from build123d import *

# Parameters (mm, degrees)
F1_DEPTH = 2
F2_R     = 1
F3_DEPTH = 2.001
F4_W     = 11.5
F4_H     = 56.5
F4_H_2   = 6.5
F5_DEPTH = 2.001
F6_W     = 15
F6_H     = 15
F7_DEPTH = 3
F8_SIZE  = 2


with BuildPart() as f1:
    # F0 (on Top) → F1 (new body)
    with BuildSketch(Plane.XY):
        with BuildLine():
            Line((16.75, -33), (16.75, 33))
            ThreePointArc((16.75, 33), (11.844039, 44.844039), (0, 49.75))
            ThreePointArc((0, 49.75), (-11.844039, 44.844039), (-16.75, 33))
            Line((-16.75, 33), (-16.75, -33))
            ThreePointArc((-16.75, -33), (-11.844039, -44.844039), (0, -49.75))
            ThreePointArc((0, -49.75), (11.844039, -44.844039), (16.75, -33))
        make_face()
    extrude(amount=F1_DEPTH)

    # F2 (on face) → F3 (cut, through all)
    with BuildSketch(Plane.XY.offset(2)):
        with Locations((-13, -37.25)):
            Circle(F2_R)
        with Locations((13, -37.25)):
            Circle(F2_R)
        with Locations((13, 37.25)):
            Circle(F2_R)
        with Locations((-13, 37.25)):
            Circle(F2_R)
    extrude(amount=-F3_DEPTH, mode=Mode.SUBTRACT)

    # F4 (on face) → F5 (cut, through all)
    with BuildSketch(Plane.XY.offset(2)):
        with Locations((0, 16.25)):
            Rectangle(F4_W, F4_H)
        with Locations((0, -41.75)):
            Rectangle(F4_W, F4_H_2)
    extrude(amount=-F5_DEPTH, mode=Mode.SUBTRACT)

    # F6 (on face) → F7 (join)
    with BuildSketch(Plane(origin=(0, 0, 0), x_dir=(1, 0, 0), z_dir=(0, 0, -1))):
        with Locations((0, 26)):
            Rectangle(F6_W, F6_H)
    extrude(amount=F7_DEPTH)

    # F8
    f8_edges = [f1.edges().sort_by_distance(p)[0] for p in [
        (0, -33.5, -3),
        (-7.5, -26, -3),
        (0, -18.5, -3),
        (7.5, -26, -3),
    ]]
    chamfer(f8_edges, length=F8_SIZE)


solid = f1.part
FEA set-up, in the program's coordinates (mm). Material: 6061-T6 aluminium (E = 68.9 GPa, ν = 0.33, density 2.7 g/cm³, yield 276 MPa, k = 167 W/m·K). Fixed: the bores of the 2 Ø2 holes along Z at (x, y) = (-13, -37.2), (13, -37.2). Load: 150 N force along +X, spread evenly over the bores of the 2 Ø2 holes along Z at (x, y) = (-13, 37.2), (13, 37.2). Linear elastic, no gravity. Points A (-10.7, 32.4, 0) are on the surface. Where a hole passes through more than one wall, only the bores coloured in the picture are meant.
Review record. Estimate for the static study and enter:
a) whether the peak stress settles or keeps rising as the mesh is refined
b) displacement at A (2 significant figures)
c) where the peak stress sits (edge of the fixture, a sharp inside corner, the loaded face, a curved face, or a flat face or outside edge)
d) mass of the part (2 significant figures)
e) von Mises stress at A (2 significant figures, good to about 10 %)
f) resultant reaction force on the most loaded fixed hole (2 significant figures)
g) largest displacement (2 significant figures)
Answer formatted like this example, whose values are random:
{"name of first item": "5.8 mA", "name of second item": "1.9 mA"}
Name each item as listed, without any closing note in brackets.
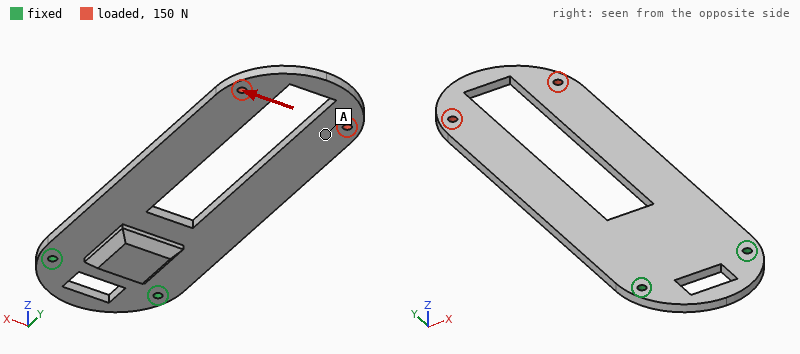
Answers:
{"whether the peak stress settles or keeps rising as the mesh is refined": "keeps rising", "displacement at A": "0.19 mm", "where the peak stress sits": "a sharp inside corner", "mass of the part": "14 g", "von Mises stress at A": "9.8 MPa", "resultant reaction force on the most loaded fixed hole": "430 N", "largest displacement": "0.24 mm"}
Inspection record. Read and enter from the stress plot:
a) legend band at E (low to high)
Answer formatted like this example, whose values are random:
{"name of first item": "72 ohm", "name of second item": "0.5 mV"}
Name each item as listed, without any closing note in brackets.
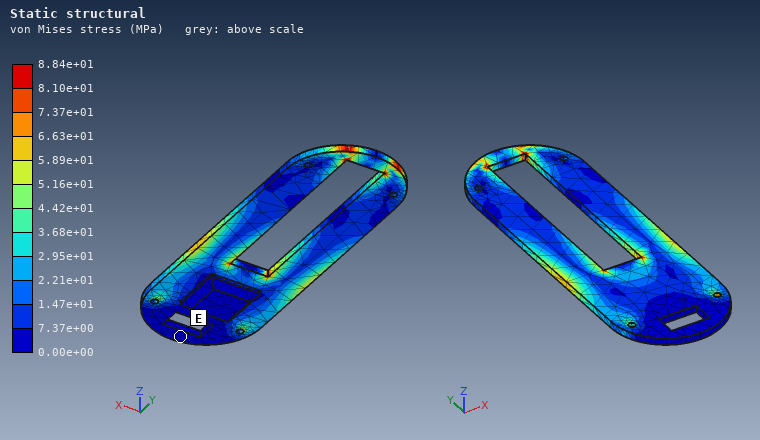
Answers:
{"legend band at E": "0.00e+00 to 7.37e+00 MPa"}
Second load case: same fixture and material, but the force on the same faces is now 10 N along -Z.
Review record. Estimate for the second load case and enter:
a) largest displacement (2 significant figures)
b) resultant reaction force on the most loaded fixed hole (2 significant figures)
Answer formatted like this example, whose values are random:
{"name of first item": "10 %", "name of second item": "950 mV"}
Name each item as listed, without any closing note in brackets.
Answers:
{"largest displacement": "1.2 mm", "resultant reaction force on the most loaded fixed hole": "5.3 N"}
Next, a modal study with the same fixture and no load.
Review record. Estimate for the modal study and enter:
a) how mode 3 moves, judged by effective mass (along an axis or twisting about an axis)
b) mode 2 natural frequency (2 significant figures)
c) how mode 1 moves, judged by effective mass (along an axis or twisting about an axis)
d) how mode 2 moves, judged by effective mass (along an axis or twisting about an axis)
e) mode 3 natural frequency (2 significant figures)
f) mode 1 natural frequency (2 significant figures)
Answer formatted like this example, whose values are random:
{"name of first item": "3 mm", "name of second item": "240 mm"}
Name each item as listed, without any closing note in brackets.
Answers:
{"how mode 3 moves, judged by effective mass": "along Z", "mode 2 natural frequency": "1100 Hz", "how mode 1 moves, judged by effective mass": "along Z", "how mode 2 moves, judged by effective mass": "twisting about Y", "mode 3 natural frequency": "1400 Hz", "mode 1 natural frequency": "290 Hz"}
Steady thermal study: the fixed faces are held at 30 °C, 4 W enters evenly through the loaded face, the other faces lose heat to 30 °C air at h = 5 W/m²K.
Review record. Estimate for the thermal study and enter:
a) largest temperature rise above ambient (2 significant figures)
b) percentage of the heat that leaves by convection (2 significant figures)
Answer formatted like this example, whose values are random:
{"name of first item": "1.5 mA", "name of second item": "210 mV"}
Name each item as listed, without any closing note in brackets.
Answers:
{"largest temperature rise above ambient": "36 K", "percentage of the heat that leaves by convection": "11 %"}
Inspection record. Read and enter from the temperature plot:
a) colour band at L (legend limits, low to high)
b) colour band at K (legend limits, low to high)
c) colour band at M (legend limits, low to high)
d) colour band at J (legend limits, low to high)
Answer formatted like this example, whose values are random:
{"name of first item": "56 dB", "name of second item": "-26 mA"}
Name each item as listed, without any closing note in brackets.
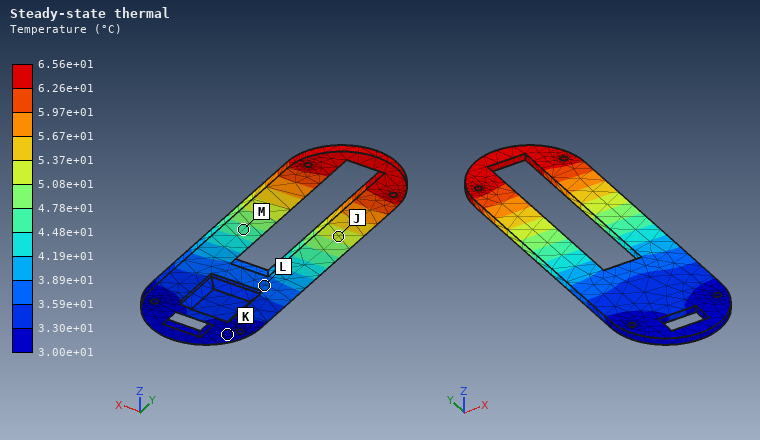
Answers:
{"colour band at L": "3.59e+01 to 3.89e+01 °C", "colour band at K": "3.00e+01 to 3.30e+01 °C", "colour band at M": "4.48e+01 to 4.78e+01 °C", "colour band at J": "5.08e+01 to 5.37e+01 °C"}
